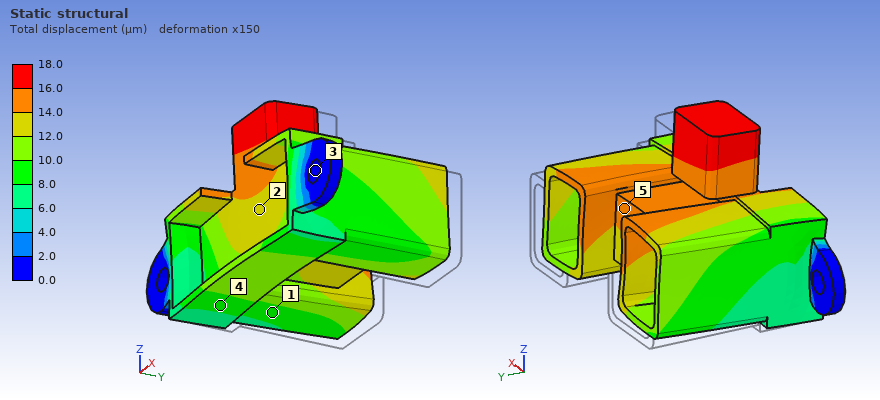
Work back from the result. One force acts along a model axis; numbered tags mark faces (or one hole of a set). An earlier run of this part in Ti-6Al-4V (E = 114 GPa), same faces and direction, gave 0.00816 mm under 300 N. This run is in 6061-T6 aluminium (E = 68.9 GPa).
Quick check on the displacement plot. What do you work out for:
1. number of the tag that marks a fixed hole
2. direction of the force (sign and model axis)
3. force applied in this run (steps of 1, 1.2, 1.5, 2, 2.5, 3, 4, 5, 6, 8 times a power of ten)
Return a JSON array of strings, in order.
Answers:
["3", "-Y", "400 N"]
